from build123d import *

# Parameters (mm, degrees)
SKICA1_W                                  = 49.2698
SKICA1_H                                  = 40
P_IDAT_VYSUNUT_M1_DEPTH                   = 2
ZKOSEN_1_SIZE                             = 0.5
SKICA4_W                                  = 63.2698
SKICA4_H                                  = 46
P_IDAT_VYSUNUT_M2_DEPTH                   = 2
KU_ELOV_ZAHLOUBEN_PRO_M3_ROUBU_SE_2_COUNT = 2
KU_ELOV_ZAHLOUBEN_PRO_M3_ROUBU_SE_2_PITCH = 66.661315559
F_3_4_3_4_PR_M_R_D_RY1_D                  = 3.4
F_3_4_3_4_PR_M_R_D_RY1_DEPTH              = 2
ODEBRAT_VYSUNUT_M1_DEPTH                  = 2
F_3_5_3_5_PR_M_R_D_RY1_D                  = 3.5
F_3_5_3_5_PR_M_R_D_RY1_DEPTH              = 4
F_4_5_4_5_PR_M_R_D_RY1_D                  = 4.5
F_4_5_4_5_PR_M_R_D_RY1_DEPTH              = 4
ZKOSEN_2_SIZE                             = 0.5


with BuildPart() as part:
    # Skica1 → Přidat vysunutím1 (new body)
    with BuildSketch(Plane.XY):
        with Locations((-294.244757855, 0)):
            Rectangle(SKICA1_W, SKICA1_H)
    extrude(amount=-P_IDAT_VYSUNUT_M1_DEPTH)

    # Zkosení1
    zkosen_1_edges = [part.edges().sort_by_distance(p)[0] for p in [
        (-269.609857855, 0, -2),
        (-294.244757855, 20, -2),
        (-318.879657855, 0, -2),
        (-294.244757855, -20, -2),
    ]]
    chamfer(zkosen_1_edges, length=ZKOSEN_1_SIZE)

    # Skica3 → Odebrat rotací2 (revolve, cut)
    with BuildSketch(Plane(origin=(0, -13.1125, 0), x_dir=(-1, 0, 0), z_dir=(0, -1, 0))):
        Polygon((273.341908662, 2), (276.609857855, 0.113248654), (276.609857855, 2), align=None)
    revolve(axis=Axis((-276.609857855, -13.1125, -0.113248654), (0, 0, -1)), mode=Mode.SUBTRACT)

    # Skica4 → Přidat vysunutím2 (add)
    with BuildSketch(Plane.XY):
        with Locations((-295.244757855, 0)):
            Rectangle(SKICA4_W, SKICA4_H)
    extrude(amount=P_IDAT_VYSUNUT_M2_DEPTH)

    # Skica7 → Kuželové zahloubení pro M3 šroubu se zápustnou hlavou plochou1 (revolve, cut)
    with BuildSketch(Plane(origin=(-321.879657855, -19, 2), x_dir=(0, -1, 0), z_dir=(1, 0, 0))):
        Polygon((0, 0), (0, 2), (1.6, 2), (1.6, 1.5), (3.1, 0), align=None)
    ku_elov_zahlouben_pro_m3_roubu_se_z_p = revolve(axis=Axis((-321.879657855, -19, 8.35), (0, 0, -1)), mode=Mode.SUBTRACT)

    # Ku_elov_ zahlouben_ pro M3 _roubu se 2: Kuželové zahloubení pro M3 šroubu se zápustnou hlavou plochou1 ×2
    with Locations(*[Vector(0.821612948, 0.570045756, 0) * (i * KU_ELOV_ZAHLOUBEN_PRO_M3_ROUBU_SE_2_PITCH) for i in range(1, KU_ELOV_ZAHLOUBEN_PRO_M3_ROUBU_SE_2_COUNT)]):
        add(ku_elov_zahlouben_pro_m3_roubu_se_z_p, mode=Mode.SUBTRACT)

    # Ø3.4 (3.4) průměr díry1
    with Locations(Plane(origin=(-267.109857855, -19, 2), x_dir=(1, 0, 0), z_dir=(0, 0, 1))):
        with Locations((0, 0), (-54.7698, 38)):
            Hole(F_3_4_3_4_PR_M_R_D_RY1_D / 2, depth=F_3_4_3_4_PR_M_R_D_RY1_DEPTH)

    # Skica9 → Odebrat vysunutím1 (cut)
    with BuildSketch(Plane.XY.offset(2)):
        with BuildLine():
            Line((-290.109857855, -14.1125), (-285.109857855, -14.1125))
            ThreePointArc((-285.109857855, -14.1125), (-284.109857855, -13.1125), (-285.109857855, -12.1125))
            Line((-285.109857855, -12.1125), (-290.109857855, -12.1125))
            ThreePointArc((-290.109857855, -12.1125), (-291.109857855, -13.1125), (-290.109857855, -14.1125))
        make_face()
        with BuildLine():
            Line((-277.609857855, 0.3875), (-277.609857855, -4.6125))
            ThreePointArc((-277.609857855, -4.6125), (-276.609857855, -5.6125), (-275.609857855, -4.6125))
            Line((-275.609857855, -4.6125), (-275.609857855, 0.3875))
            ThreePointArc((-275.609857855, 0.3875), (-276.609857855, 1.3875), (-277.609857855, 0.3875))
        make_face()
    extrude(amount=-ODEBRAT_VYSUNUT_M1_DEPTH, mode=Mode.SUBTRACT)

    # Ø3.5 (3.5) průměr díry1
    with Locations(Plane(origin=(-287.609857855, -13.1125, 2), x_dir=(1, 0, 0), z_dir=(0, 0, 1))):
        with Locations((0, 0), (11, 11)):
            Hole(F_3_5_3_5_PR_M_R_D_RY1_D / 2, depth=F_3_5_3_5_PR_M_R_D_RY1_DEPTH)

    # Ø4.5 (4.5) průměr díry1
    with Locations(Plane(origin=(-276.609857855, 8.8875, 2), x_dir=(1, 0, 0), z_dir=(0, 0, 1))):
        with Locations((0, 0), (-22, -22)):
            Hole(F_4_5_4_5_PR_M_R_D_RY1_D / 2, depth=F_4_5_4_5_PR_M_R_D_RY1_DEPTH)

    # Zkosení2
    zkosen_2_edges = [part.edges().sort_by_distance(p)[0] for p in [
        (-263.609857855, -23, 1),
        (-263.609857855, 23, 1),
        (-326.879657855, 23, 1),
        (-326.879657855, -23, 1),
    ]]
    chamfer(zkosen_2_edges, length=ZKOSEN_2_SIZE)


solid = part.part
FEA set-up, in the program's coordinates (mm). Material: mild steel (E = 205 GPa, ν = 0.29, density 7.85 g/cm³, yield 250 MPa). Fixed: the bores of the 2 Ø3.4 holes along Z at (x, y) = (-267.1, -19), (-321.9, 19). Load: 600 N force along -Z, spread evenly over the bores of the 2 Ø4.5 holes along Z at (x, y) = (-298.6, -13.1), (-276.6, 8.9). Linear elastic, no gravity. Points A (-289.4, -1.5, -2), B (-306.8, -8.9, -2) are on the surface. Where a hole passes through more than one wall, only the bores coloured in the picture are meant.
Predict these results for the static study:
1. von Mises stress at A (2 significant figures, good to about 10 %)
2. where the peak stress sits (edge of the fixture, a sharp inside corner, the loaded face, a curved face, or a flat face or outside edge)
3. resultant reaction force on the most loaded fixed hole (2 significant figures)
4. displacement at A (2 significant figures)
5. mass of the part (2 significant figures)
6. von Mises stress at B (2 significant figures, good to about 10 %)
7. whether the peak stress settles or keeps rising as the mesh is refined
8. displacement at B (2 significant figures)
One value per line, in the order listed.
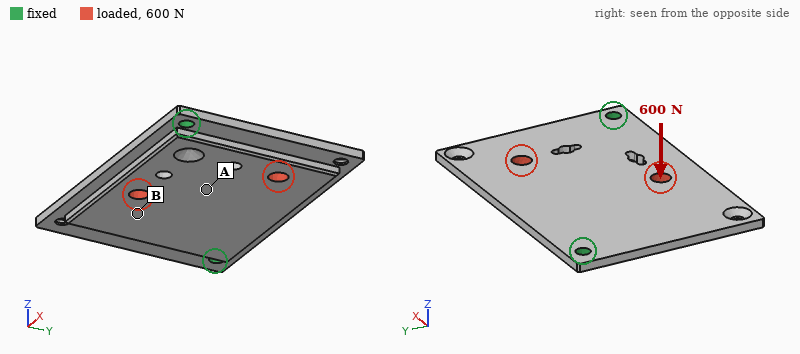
71 MPa
edge of the fixture
900 N
0.053 mm
74 g
31 MPa
keeps rising
0.040 mm
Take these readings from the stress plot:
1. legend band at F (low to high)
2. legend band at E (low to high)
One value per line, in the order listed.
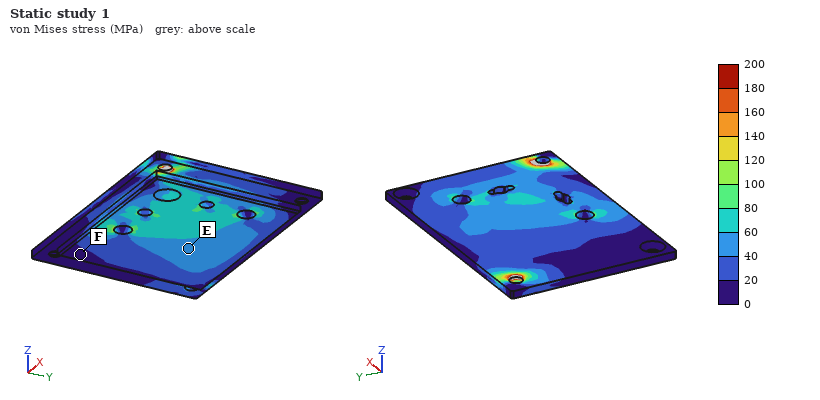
0 to 20 MPa
40 to 60 MPa
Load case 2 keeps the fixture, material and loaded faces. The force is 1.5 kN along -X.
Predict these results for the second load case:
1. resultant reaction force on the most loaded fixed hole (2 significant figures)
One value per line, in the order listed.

780 N
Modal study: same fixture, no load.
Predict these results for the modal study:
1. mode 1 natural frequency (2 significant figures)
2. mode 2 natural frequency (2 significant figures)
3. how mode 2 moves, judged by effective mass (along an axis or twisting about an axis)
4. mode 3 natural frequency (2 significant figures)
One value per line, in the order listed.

1500 Hz
2300 Hz
along Z
6100 Hz
